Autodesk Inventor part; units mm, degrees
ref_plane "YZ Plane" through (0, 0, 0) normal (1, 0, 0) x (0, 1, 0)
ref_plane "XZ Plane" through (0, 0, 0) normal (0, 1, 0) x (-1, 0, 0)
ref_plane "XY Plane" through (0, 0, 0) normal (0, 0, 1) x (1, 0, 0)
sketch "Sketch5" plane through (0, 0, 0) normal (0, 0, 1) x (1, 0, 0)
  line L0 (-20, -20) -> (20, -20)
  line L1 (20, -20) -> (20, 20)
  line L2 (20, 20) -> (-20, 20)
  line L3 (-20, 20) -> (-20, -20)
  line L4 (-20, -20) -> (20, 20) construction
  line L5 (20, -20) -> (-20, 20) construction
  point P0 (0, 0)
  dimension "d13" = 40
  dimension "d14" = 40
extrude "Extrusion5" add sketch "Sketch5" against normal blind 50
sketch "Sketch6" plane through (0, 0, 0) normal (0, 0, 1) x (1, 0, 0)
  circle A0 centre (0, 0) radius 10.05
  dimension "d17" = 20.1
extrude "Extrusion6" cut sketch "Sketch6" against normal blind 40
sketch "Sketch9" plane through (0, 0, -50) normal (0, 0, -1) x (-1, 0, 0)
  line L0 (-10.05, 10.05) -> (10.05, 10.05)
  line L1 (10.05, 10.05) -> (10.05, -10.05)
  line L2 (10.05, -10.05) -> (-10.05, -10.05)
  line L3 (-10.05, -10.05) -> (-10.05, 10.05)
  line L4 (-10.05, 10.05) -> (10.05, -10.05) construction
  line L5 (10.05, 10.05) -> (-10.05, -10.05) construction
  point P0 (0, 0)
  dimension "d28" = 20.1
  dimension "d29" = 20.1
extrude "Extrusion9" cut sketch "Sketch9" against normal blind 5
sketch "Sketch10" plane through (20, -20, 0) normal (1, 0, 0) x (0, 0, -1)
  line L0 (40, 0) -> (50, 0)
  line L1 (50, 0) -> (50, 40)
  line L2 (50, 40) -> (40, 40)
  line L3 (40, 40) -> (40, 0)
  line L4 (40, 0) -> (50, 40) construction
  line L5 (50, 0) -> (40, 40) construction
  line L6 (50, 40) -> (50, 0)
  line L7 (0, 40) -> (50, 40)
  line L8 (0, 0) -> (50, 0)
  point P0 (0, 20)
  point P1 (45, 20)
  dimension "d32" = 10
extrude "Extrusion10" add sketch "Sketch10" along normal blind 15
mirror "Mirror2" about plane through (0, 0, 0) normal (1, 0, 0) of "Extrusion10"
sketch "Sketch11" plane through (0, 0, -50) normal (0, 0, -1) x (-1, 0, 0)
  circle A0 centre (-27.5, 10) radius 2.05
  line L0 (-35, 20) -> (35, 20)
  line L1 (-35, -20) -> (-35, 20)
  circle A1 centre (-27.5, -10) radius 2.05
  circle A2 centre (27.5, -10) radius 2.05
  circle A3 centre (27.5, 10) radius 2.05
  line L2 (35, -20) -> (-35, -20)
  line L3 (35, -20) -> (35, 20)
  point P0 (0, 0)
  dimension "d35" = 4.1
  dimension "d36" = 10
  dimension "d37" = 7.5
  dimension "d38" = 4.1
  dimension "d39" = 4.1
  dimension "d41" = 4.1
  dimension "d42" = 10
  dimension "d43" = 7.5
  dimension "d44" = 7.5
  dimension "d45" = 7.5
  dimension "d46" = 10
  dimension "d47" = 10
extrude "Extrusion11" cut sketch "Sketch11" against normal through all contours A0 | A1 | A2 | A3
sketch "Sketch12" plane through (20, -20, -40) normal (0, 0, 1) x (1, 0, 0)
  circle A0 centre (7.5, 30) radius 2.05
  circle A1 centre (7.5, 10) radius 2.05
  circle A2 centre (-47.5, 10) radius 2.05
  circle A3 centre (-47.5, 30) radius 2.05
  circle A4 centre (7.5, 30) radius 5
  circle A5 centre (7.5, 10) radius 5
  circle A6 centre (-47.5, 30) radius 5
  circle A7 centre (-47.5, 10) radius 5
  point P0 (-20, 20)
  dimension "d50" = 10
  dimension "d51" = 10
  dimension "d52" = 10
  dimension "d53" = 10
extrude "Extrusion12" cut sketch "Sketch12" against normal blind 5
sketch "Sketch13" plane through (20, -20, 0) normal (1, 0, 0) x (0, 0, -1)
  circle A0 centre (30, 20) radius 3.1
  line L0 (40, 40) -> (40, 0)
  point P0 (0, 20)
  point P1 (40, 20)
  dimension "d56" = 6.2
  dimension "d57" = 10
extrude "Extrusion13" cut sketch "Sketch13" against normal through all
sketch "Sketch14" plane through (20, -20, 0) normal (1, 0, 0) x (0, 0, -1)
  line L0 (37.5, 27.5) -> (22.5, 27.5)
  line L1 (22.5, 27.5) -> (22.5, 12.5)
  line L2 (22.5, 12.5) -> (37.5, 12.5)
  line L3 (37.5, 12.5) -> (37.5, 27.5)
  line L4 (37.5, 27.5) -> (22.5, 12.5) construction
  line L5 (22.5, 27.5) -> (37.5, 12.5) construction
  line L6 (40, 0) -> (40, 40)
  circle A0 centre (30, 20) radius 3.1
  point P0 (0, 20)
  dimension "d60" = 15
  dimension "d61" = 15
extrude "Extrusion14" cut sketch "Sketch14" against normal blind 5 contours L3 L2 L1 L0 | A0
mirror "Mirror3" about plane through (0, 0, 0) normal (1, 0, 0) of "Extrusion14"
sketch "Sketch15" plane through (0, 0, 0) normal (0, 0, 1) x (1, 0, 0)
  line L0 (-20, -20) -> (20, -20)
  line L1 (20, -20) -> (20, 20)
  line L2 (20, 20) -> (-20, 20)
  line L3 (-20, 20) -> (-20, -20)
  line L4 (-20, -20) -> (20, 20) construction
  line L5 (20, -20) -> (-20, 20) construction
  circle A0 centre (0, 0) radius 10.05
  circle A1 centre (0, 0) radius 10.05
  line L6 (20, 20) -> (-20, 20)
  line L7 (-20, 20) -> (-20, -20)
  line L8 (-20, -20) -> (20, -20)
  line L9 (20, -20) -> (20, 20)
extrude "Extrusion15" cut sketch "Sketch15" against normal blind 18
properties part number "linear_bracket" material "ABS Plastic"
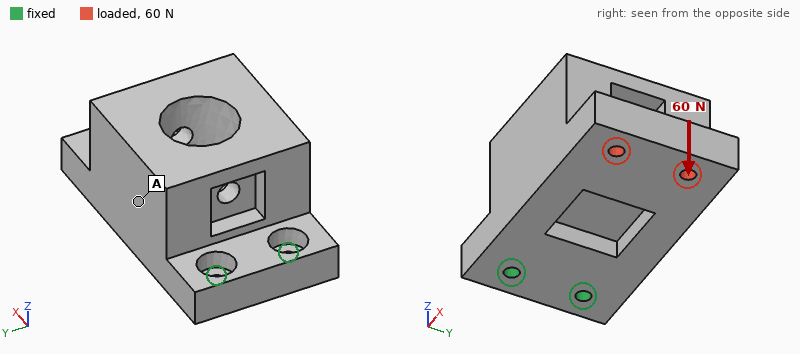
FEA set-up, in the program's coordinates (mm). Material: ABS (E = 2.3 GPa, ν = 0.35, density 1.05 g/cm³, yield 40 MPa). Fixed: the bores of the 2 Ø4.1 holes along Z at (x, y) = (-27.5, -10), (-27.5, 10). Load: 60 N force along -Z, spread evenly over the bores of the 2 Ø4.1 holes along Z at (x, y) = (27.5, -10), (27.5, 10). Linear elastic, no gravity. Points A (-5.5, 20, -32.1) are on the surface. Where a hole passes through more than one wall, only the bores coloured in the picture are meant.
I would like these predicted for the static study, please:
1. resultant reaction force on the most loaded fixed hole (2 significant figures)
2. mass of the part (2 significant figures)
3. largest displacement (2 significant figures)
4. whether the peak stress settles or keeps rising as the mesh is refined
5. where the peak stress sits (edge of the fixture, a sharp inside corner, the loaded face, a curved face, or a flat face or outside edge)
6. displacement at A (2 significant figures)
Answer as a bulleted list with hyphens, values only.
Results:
- 32 N
- 52 g
- 0.86 mm
- keeps rising
- edge of the fixture
- 0.33 mm
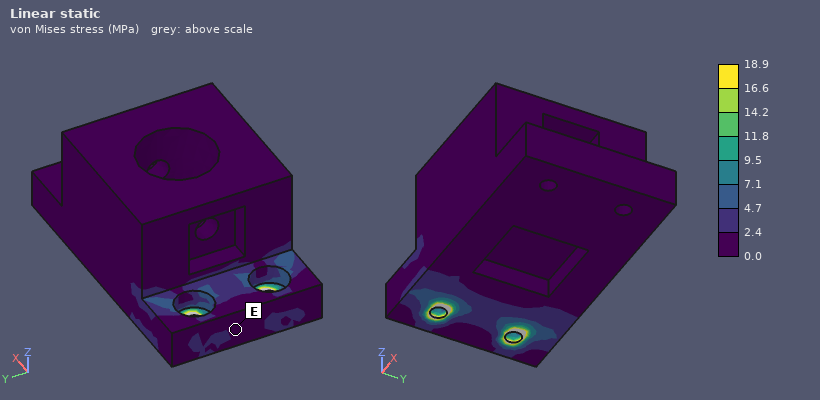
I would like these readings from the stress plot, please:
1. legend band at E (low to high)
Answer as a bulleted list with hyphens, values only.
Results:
- 0.0 to 2.4 MPa
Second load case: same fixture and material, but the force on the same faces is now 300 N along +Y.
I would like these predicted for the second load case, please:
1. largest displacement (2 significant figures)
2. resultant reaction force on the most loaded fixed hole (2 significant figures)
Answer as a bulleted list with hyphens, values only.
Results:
- 0.50 mm
- 740 N
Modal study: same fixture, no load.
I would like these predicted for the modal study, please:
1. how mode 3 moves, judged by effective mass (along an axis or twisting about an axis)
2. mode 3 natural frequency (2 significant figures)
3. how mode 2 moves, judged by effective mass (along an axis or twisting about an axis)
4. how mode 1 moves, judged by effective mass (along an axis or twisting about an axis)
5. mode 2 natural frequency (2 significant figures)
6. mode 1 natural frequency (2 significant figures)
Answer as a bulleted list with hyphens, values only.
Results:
- twisting about X
- 1300 Hz
- along Y
- along Z
- 1100 Hz
- 320 Hz
